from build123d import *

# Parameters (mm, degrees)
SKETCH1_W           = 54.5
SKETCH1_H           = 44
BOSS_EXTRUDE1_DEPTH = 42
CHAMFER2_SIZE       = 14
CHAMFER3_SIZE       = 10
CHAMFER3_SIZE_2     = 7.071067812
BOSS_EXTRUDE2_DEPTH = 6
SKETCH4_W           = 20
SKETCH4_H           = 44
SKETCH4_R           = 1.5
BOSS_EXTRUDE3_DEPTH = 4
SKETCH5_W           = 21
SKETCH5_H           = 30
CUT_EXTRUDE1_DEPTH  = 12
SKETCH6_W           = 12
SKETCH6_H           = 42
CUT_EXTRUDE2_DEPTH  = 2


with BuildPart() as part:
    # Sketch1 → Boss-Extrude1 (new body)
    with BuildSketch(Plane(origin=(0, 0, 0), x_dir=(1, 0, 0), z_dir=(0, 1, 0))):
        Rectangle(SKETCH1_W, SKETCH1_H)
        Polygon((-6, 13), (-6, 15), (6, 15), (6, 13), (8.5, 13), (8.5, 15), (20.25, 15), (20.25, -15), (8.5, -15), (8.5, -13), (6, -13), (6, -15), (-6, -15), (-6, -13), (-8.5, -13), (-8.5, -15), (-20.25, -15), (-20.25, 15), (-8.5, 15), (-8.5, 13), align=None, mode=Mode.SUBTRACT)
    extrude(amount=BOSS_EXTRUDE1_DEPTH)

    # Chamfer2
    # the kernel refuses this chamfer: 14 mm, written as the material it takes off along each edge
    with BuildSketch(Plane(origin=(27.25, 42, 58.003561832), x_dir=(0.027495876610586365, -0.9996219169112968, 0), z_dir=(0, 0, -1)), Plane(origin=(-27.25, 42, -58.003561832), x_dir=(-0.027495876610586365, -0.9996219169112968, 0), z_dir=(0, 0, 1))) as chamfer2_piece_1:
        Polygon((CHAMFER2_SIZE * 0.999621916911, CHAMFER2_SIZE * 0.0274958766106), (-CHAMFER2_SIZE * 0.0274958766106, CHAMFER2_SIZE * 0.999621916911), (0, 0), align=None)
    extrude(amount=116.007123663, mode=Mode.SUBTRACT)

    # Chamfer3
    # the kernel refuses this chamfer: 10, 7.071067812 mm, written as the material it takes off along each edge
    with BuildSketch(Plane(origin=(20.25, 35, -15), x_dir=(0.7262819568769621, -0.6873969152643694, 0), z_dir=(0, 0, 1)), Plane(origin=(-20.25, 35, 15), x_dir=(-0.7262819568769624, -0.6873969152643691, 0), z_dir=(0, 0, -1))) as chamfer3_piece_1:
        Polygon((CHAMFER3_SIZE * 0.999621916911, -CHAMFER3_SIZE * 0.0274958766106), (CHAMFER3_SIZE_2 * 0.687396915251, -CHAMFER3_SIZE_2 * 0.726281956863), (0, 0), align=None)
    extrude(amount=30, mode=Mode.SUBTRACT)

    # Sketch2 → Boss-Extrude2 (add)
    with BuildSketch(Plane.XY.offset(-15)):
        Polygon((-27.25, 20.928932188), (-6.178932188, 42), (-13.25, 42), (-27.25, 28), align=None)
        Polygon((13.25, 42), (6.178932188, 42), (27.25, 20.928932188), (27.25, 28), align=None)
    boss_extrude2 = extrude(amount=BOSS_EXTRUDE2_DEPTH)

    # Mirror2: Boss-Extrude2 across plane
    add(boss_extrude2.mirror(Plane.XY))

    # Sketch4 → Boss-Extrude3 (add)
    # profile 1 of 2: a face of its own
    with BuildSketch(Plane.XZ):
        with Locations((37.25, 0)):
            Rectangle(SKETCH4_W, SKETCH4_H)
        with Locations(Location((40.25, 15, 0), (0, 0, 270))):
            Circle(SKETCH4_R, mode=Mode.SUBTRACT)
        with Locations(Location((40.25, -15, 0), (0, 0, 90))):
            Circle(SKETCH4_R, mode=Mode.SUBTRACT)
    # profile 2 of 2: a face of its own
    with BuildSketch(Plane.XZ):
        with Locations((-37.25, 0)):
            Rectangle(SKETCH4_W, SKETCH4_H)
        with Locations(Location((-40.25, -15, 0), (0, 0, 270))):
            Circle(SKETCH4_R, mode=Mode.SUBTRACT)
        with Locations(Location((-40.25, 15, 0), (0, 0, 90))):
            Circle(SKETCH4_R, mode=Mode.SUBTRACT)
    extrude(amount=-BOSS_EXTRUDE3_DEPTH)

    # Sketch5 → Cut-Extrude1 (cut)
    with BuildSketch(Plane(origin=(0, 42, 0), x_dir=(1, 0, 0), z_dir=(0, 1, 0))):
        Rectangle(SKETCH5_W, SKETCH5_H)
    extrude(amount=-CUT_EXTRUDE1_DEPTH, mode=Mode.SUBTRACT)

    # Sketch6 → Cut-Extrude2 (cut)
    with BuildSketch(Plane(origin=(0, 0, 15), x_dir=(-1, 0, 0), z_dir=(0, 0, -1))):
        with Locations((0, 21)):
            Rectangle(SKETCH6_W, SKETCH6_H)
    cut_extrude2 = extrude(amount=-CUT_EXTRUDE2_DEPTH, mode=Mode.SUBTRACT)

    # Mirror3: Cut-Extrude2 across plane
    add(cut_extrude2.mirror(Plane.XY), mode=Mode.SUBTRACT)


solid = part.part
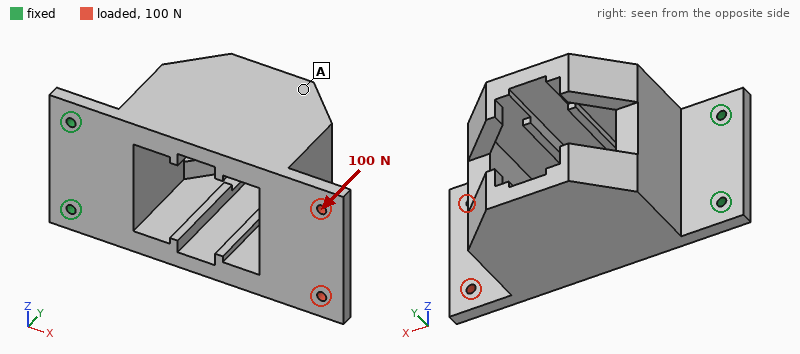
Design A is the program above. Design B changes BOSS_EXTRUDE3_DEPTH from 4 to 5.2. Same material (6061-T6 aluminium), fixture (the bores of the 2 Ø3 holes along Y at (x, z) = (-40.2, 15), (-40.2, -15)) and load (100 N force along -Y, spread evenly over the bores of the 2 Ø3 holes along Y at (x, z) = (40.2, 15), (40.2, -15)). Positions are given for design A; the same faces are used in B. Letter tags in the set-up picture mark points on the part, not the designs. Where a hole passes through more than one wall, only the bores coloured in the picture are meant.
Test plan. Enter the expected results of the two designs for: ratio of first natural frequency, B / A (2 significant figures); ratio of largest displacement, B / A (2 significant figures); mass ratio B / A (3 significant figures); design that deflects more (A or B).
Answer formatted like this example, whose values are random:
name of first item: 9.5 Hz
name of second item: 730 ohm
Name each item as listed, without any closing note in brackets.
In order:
ratio of first natural frequency, B / A: 1.4
ratio of largest displacement, B / A: 0.51
mass ratio B / A: 1.04
design that deflects more: A
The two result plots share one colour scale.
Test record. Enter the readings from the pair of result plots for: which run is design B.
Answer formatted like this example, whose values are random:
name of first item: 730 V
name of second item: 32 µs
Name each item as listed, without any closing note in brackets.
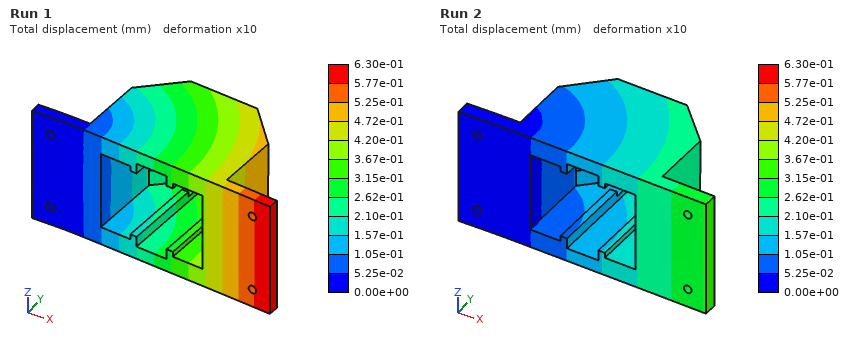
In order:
which run is design B: Run 2
